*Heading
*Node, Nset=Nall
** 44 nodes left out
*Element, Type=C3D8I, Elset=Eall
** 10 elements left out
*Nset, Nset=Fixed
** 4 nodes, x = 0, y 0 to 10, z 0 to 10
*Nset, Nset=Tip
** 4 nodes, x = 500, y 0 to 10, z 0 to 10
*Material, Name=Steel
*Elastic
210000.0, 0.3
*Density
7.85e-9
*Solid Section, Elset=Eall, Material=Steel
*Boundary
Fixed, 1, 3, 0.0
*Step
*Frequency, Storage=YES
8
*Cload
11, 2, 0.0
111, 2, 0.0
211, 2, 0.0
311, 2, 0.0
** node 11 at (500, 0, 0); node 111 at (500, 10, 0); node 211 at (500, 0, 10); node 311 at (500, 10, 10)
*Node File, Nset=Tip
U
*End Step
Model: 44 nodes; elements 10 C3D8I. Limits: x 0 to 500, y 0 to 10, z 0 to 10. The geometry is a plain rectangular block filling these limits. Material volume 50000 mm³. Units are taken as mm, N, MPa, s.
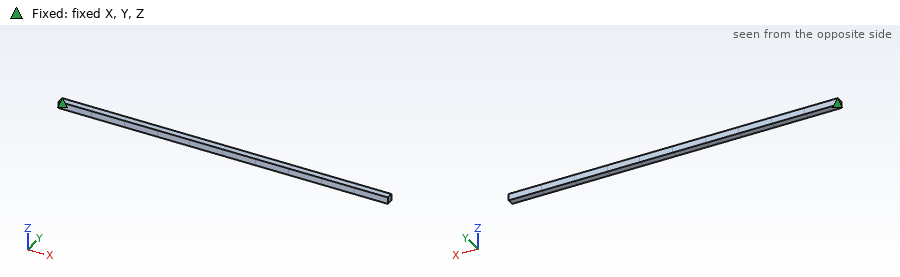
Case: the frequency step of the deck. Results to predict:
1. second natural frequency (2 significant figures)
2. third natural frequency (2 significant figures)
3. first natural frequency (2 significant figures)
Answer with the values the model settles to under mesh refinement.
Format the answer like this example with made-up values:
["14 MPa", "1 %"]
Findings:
["34 Hz", "210 Hz", "34 Hz"]
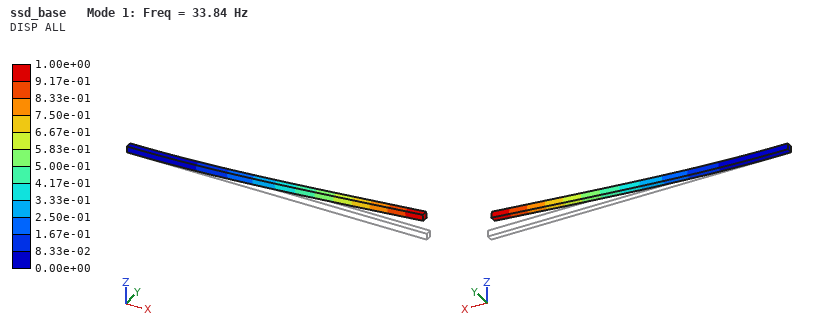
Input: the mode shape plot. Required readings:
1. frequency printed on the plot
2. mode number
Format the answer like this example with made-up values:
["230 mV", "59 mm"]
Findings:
["33.84 Hz", "1"]
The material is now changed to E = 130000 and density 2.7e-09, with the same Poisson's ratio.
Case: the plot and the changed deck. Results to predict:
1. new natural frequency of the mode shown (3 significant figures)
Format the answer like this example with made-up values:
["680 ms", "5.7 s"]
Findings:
["45.4 Hz"]
